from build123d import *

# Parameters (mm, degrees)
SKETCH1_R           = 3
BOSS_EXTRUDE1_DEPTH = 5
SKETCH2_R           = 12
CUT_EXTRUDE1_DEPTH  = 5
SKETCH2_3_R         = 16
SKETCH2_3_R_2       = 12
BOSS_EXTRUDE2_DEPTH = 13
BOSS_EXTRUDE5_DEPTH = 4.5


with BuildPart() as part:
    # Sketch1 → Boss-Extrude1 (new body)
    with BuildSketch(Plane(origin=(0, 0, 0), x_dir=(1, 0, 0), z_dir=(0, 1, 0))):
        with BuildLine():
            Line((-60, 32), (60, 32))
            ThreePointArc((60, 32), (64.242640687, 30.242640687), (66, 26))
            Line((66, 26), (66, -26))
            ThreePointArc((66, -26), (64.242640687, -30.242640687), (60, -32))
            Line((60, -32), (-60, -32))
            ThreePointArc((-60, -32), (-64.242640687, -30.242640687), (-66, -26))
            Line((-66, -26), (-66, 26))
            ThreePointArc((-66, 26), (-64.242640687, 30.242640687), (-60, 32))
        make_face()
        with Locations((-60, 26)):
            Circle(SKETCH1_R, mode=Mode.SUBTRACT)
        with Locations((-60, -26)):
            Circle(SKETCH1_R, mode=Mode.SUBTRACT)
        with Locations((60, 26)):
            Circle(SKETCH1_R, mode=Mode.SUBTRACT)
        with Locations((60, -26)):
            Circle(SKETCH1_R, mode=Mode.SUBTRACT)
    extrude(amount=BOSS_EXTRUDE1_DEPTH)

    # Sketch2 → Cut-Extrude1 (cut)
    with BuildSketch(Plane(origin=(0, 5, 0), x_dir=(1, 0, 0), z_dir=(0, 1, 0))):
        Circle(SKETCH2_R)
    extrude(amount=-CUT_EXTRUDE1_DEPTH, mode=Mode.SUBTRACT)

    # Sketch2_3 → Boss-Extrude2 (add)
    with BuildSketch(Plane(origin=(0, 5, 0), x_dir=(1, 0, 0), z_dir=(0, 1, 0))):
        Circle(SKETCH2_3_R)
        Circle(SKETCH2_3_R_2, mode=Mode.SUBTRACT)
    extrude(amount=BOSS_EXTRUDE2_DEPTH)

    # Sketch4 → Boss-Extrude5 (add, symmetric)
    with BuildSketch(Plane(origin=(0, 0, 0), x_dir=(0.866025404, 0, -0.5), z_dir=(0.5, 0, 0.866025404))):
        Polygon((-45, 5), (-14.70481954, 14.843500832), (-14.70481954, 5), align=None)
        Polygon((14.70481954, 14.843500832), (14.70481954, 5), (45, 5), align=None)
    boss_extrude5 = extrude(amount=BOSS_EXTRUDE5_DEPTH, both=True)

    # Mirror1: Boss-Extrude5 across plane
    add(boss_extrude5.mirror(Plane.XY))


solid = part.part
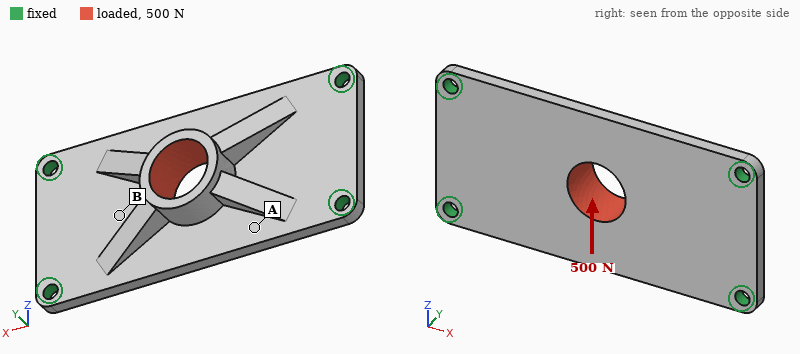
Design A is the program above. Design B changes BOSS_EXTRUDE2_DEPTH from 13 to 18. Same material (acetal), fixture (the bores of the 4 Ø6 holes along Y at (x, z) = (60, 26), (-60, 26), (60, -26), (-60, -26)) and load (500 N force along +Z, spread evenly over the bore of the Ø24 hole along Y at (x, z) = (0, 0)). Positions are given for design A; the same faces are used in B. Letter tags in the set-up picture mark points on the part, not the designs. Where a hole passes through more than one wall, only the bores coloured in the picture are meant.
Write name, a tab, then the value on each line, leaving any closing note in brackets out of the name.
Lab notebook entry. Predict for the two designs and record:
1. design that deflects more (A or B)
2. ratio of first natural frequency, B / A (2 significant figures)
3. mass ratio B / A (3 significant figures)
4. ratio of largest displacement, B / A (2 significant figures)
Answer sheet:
design that deflects more	B
ratio of first natural frequency, B / A	1.00
mass ratio B / A	1.04
ratio of largest displacement, B / A	1.4
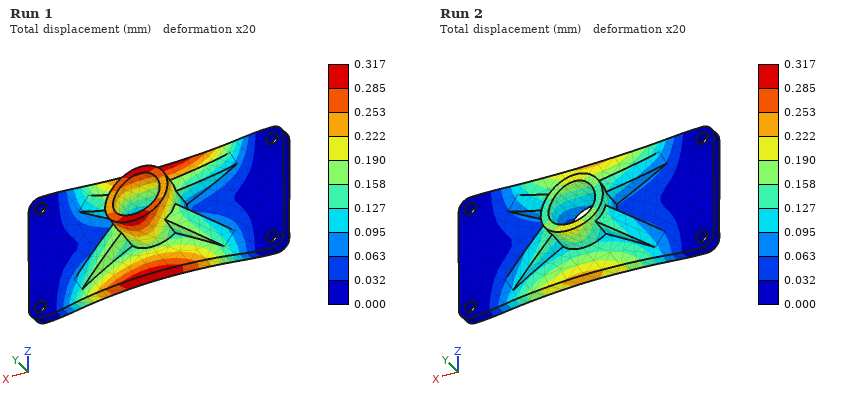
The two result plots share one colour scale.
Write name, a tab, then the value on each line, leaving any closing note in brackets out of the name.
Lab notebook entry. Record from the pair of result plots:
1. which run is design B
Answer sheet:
which run is design B	Run 1
